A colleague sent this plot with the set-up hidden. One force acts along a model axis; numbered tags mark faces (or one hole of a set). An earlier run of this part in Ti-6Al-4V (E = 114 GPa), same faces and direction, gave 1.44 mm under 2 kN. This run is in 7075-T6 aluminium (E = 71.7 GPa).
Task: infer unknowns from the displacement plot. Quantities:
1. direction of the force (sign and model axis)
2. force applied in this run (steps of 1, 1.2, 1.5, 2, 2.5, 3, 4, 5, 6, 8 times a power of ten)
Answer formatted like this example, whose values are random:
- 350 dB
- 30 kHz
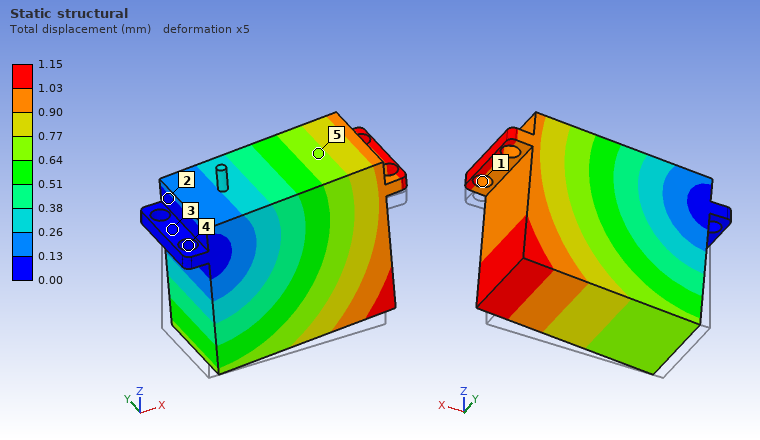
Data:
- +Z
- 1 kN
